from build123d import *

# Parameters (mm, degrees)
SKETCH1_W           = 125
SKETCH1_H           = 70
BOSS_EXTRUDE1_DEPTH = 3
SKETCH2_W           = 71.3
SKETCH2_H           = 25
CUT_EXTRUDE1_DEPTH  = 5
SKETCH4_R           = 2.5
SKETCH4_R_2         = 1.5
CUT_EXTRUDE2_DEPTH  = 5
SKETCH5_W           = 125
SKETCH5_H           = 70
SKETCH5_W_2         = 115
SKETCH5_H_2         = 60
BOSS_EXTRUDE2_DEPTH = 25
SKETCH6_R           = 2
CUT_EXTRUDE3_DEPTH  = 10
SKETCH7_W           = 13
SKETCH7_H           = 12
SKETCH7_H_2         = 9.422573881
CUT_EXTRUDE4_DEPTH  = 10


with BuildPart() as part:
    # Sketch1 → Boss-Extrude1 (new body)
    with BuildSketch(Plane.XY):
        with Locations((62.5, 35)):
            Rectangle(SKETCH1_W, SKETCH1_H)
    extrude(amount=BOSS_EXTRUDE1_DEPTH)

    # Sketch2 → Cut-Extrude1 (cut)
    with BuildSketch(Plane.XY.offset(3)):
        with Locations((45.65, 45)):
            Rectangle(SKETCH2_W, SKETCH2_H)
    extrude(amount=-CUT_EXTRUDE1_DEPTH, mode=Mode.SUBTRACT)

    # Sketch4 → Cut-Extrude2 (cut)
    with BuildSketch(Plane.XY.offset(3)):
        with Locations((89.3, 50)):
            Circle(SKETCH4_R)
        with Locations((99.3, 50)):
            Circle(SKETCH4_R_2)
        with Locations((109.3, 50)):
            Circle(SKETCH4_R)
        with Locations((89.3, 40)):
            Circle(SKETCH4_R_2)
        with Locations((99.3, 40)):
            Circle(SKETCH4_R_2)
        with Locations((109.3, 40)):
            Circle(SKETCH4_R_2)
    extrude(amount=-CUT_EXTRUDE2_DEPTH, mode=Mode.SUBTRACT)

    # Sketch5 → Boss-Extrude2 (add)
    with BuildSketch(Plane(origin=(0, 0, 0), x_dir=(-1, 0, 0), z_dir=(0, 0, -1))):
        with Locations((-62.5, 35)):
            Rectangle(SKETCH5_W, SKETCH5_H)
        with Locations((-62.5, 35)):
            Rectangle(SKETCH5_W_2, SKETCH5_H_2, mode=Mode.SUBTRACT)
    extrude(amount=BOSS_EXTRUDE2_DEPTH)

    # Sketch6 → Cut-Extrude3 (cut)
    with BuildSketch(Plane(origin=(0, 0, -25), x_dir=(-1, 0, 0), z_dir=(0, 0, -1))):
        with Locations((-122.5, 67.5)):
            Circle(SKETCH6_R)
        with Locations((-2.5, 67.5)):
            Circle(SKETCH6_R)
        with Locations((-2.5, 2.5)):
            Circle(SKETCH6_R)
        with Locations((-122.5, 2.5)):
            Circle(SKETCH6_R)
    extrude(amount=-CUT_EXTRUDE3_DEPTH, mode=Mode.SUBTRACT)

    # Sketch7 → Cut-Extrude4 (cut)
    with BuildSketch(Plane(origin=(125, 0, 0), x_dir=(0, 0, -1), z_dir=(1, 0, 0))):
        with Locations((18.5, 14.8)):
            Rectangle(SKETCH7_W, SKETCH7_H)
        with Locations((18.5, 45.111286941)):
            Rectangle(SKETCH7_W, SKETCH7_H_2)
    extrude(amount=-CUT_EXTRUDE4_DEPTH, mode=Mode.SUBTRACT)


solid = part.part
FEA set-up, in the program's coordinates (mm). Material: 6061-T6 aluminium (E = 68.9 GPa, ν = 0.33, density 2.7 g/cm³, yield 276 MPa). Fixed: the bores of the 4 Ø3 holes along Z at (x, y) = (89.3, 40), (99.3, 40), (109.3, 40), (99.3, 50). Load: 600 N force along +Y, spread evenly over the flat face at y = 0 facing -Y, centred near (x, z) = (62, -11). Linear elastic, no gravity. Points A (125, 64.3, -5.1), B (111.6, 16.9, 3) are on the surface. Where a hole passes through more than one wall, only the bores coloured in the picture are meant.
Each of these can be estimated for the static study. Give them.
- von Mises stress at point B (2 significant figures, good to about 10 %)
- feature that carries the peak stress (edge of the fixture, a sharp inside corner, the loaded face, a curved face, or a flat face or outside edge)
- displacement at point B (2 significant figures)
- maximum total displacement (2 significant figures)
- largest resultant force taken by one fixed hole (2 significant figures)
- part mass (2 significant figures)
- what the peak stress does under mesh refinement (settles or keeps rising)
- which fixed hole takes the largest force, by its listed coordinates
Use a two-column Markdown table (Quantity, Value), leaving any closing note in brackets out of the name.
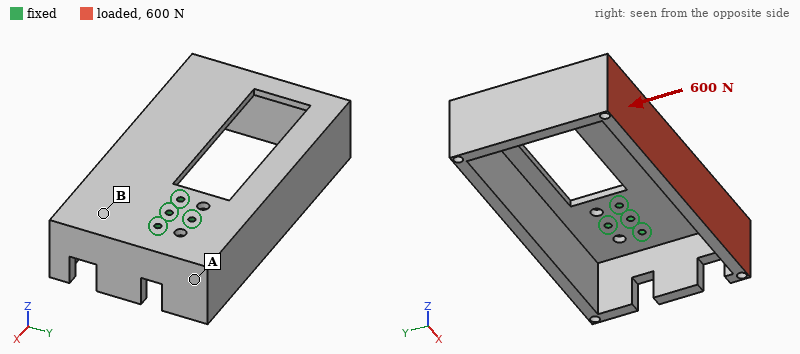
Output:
| Quantity | Value |
|---|---|
| von Mises stress at point B | 21 MPa |
| feature that carries the peak stress | edge of the fixture |
| displacement at point B | 0.075 mm |
| maximum total displacement | 0.44 mm |
| largest resultant force taken by one fixed hole | 1.1 kN |
| part mass | 180 g |
| what the peak stress does under mesh refinement | keeps rising |
| which fixed hole takes the largest force, by its listed coordinates | (89.3, 40) |
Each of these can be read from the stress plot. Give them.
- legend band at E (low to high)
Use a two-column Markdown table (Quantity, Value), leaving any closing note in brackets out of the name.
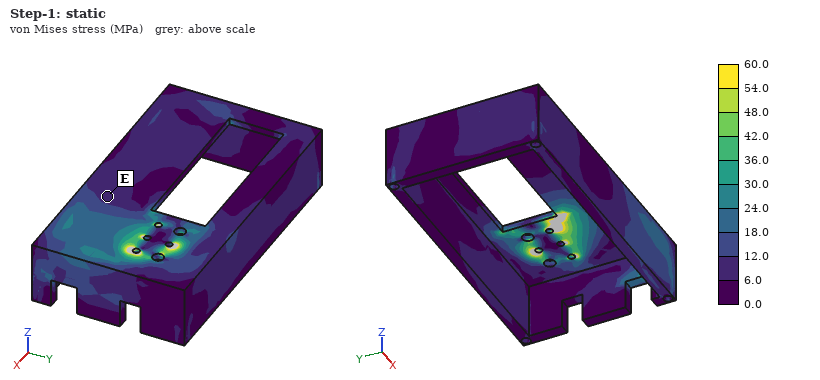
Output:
| Quantity | Value |
|---|---|
| legend band at E | 6.0 to 12.0 MPa |
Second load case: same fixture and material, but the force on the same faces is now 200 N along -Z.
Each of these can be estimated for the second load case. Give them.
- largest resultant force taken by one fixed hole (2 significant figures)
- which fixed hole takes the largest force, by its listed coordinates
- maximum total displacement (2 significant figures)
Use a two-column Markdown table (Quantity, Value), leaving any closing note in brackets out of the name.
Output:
| Quantity | Value |
|---|---|
| largest resultant force taken by one fixed hole | 350 N |
| which fixed hole takes the largest force, by its listed coordinates | (89.3, 40) |
| maximum total displacement | 0.81 mm |
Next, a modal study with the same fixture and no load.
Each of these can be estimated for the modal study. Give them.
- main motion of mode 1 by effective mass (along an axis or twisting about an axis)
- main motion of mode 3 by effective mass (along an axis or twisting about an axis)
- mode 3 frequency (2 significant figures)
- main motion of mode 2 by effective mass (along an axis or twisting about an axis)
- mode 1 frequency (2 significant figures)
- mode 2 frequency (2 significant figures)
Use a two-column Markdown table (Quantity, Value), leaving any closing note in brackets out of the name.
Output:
| Quantity | Value |
|---|---|
| main motion of mode 1 by effective mass | along Z |
| main motion of mode 3 by effective mass | along Y |
| mode 3 frequency | 1200 Hz |
| main motion of mode 2 by effective mass | along Y |
| mode 1 frequency | 290 Hz |
| mode 2 frequency | 590 Hz |
